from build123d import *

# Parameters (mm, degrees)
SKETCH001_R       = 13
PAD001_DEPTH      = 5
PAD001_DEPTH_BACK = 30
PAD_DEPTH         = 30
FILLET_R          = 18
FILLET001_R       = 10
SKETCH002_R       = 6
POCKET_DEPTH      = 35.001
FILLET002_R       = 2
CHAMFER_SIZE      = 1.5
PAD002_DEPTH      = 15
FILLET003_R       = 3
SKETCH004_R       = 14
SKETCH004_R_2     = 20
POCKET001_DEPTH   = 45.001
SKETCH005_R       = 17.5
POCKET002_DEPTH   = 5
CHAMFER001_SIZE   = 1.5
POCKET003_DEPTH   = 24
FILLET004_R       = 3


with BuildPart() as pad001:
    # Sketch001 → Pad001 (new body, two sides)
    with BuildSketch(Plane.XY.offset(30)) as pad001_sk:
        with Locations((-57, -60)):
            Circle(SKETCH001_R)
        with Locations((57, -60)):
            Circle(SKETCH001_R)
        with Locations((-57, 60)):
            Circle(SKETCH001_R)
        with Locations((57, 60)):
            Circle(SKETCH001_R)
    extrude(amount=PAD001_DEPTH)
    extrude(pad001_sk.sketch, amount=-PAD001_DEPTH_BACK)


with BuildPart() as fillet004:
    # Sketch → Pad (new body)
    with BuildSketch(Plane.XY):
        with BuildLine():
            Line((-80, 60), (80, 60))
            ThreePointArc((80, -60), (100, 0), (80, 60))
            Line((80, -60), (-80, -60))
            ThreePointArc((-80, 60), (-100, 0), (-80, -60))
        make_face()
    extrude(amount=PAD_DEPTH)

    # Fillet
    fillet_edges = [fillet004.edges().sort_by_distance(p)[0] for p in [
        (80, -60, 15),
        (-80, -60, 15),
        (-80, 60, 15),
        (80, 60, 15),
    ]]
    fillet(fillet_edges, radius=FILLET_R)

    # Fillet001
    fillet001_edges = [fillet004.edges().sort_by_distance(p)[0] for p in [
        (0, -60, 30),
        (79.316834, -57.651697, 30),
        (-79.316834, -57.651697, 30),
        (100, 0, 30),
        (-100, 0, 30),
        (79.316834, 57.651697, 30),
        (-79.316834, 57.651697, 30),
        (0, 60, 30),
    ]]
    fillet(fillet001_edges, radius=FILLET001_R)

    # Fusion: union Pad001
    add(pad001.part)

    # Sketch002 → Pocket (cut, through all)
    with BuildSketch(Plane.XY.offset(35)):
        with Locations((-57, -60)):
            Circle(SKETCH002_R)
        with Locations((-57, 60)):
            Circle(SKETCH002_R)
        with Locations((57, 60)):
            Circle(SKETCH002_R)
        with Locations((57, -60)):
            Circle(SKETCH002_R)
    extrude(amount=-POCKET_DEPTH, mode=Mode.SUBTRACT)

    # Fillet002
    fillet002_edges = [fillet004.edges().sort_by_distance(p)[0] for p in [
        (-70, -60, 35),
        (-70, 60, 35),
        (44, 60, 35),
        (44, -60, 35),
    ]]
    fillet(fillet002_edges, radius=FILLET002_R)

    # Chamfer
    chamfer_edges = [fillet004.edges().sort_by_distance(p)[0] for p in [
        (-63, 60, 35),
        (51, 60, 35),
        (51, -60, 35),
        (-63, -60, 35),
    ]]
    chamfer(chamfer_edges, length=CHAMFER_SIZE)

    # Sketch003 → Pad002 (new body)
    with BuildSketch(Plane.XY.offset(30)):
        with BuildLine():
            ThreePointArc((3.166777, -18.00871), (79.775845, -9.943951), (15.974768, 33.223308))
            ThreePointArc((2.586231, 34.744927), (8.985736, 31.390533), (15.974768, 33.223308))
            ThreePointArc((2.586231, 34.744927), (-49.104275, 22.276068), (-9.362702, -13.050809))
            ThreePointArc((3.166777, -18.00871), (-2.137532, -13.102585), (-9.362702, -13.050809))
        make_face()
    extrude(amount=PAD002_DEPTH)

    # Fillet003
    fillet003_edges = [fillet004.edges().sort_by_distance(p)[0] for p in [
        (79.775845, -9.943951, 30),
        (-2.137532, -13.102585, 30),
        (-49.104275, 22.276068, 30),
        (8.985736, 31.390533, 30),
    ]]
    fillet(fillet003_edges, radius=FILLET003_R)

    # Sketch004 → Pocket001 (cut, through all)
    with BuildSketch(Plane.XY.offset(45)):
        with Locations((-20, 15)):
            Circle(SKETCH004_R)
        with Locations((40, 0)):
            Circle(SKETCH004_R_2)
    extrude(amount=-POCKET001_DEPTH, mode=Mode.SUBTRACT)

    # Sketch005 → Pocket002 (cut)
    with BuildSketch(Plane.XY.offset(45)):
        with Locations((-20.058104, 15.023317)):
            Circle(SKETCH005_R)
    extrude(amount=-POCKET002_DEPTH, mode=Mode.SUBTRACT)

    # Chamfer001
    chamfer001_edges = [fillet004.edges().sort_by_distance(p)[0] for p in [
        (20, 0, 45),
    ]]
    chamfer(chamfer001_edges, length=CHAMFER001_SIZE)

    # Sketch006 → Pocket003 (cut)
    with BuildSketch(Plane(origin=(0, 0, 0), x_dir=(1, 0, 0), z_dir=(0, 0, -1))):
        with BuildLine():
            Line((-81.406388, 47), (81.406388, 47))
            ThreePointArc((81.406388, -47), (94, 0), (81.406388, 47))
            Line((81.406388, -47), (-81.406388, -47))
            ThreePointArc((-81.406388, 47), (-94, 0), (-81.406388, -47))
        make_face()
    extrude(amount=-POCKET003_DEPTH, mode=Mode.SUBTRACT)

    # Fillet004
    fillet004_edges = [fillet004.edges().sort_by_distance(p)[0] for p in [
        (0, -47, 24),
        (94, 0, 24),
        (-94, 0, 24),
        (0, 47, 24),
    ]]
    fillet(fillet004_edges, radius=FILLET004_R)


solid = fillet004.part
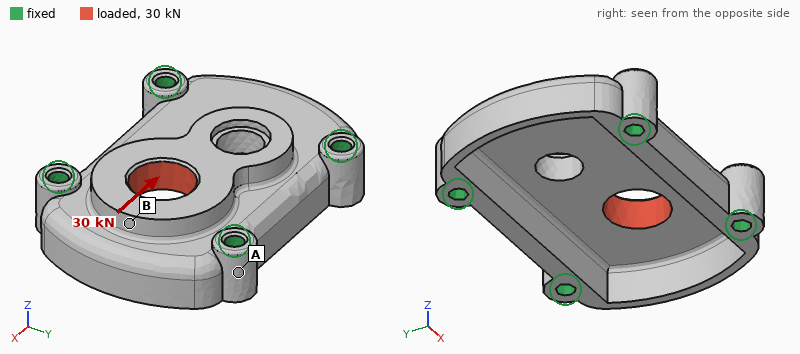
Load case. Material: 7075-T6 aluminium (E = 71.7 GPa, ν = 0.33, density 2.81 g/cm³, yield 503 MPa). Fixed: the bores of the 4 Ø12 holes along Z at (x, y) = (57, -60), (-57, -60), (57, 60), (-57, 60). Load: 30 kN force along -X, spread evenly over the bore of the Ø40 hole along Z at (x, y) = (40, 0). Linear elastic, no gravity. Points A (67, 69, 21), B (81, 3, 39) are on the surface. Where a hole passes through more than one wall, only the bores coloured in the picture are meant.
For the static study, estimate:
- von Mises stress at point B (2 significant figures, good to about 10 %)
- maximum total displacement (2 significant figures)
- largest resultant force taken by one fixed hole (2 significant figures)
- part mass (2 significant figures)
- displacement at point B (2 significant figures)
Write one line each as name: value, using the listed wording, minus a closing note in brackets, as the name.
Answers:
von Mises stress at point B: 15 MPa
maximum total displacement: 37 µm
largest resultant force taken by one fixed hole: 9.2 kN
part mass: 1.0 kg
displacement at point B: 34 µm
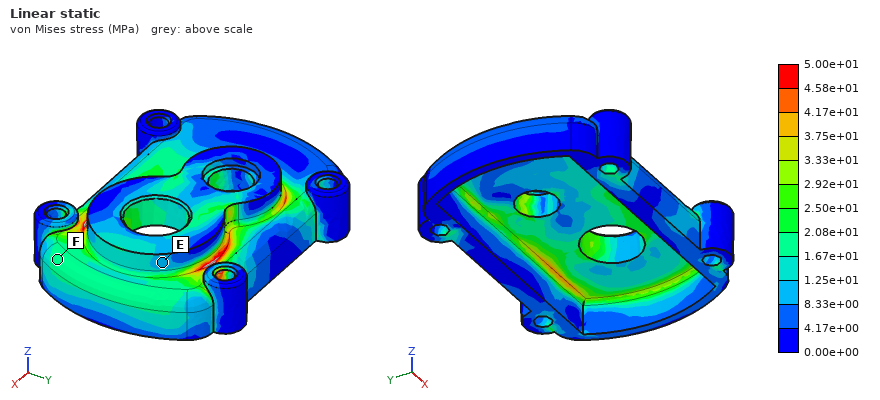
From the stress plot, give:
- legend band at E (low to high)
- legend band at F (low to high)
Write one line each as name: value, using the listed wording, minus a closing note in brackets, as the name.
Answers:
legend band at E: 8.33e+00 to 1.25e+01 MPa
legend band at F: 1.67e+01 to 2.08e+01 MPa
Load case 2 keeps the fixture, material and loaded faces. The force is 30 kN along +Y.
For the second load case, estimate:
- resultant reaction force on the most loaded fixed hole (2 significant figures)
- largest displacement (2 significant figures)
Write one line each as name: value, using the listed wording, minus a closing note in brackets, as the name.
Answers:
resultant reaction force on the most loaded fixed hole: 12 kN
largest displacement: 28 µm
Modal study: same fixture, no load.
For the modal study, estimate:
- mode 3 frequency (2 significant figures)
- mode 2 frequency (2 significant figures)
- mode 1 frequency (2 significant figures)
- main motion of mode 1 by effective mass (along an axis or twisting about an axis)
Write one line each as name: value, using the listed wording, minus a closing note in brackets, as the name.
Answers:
mode 3 frequency: 5400 Hz
mode 2 frequency: 5200 Hz
mode 1 frequency: 4000 Hz
main motion of mode 1 by effective mass: along Z
